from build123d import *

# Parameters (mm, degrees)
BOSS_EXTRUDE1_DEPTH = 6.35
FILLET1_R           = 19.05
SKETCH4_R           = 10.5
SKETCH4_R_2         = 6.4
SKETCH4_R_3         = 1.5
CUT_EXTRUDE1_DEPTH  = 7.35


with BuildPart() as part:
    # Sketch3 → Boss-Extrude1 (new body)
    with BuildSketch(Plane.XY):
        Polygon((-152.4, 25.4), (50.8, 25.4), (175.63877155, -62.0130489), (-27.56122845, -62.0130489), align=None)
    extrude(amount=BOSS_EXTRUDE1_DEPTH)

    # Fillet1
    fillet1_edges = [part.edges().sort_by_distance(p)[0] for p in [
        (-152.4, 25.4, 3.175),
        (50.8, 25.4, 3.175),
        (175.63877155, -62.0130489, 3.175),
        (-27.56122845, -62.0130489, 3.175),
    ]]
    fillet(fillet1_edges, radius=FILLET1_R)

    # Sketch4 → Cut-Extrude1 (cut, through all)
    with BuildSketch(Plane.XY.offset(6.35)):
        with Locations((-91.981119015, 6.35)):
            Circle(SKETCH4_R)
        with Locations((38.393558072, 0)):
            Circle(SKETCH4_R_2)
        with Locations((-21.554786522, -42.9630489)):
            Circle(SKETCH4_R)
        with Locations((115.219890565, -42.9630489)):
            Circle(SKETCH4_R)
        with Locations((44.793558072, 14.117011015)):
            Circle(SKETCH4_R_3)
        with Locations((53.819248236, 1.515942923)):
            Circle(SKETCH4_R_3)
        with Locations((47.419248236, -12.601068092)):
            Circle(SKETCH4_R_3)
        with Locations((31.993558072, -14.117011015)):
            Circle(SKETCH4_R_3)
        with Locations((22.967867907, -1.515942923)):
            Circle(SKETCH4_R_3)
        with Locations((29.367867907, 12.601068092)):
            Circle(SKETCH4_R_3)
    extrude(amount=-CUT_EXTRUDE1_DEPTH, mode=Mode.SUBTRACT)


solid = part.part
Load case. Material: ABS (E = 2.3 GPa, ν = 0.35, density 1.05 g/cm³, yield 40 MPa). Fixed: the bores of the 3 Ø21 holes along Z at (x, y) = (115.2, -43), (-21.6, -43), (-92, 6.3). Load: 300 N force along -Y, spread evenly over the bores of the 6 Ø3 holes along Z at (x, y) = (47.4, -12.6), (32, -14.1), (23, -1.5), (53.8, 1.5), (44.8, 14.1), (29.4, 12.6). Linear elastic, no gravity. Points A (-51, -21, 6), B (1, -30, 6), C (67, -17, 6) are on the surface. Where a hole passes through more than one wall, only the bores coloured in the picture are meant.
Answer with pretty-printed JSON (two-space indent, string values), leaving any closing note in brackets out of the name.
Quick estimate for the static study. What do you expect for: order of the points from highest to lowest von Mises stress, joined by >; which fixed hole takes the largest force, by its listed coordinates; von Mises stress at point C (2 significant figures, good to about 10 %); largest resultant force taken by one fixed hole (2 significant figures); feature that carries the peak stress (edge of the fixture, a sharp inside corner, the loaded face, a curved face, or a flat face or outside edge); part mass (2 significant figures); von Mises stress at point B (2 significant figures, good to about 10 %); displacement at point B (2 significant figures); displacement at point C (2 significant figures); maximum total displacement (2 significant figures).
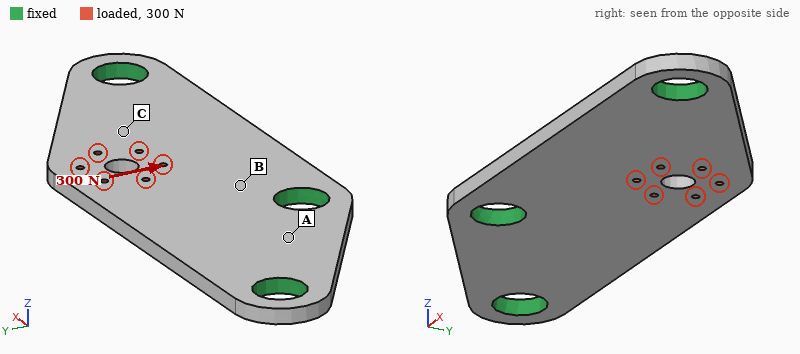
{
  "order of the points from highest to lowest von Mises stress, joined by >": "B > C > A",
  "which fixed hole takes the largest force, by its listed coordinates": "(-21.6, -43)",
  "von Mises stress at point C": "0.54 MPa",
  "largest resultant force taken by one fixed hole": "210 N",
  "feature that carries the peak stress": "the loaded face",
  "part mass": "100 g",
  "von Mises stress at point B": "0.91 MPa",
  "displacement at point B": "12 µm",
  "displacement at point C": "25 µm",
  "maximum total displacement": "36 µm"
}
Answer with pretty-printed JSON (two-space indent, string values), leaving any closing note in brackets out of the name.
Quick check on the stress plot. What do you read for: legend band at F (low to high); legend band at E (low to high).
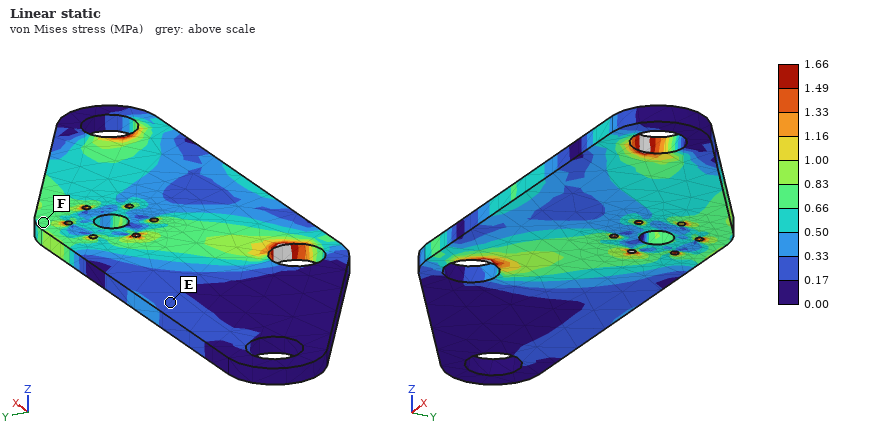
{
  "legend band at F": "0.66 to 0.83 MPa",
  "legend band at E": "0.17 to 0.33 MPa"
}
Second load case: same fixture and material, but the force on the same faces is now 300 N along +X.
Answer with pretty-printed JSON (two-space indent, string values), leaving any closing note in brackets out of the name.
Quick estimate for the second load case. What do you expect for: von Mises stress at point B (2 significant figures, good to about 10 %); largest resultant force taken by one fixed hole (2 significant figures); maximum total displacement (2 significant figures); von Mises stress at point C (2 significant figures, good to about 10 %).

{
  "von Mises stress at point B": "0.53 MPa",
  "largest resultant force taken by one fixed hole": "130 N",
  "maximum total displacement": "21 µm",
  "von Mises stress at point C": "0.48 MPa"
}
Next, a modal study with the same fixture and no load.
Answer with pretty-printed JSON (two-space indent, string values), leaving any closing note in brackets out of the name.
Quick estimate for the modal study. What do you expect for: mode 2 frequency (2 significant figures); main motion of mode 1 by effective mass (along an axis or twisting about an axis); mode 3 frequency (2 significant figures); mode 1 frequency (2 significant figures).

{
  "mode 2 frequency": "710 Hz",
  "main motion of mode 1 by effective mass": "along Z",
  "mode 3 frequency": "850 Hz",
  "mode 1 frequency": "360 Hz"
}
